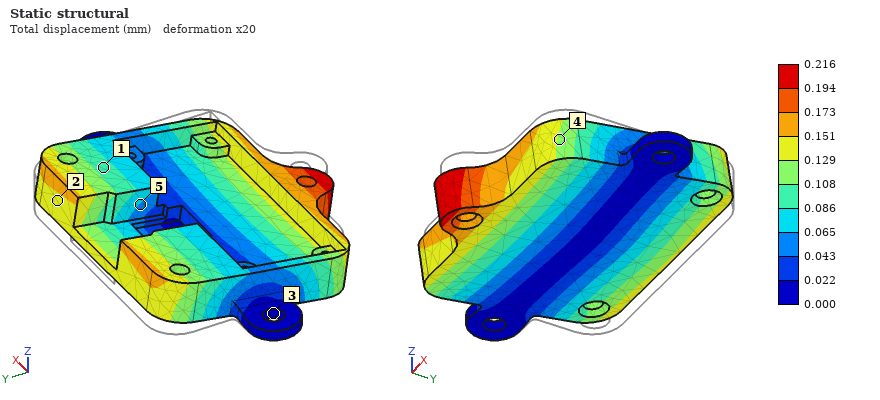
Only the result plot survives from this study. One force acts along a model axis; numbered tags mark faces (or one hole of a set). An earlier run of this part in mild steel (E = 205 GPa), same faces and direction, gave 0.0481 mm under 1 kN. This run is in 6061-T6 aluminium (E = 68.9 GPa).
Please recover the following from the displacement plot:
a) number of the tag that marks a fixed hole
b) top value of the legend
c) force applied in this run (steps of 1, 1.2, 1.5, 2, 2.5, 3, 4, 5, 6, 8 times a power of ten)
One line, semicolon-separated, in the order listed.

3; 0.216 mm; 1.5 kN
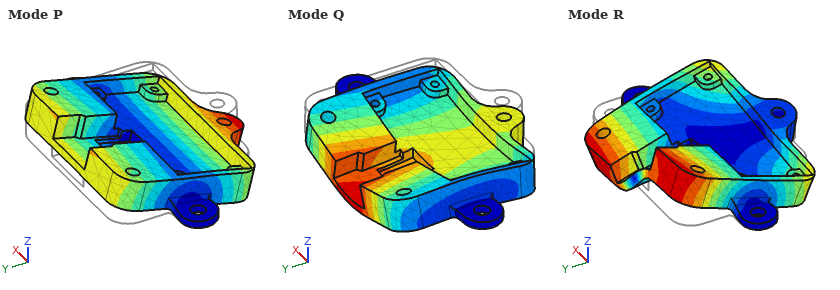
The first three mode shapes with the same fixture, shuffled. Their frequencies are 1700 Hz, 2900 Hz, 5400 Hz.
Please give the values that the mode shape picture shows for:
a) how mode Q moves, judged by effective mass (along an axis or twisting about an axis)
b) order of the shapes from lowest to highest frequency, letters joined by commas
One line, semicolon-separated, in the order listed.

along Z; P, Q, R
